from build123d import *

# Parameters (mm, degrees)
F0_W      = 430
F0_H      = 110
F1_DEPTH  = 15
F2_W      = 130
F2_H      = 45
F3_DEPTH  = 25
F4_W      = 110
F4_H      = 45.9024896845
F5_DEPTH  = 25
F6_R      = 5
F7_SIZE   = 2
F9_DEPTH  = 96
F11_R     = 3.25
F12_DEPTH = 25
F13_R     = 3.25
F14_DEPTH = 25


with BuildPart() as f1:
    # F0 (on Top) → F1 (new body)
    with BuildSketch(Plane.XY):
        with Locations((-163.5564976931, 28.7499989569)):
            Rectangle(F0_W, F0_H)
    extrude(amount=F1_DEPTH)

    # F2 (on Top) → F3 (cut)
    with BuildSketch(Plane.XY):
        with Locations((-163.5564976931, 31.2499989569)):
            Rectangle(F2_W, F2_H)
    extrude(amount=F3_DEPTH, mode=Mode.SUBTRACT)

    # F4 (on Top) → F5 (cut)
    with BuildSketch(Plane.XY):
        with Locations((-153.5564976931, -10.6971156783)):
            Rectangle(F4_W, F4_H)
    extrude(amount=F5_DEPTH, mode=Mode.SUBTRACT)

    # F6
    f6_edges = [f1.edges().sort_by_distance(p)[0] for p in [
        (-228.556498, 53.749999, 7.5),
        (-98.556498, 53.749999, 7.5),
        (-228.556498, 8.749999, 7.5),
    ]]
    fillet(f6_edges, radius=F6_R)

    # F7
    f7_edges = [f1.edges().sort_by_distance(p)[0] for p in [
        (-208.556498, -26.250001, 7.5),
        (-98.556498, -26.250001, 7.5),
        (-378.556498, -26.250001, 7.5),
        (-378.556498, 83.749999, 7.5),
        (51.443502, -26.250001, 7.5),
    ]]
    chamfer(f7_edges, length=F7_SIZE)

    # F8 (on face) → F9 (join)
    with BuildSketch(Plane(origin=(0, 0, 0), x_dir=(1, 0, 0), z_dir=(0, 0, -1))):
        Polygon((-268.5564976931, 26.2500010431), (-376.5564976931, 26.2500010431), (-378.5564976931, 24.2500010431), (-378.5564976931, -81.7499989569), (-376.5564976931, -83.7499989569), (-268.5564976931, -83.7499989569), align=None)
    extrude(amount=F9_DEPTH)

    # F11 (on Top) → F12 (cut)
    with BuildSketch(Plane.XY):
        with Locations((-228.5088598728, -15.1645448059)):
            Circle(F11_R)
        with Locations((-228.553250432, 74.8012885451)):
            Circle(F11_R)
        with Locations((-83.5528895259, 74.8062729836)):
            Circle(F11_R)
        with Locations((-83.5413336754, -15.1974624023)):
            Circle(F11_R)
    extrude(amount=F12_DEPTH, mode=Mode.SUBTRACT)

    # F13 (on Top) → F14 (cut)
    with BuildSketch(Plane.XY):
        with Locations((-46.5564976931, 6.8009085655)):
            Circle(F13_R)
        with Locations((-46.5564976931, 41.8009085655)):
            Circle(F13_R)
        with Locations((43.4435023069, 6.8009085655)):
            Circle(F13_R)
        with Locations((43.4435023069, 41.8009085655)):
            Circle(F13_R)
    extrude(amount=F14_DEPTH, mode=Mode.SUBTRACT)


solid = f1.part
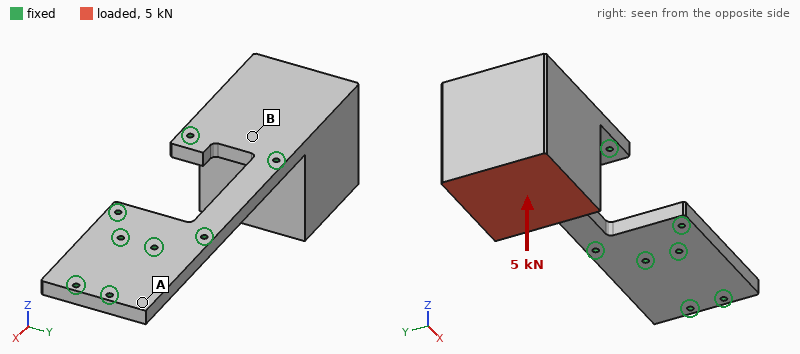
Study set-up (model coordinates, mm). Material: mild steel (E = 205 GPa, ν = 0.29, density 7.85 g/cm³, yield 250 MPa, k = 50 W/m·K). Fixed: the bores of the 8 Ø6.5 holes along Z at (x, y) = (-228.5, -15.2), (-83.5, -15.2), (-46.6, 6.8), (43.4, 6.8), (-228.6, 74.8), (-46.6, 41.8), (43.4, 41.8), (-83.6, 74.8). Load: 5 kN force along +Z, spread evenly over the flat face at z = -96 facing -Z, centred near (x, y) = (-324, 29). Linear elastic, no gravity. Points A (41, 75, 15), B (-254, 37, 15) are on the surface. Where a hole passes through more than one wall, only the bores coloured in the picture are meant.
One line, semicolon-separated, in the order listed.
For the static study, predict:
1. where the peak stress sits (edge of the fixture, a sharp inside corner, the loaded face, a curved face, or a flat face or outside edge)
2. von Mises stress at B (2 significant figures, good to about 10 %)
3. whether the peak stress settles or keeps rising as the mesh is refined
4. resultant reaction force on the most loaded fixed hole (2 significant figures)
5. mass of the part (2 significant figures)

edge of the fixture; 56 MPa; keeps rising; 2.8 kN; 14 kg
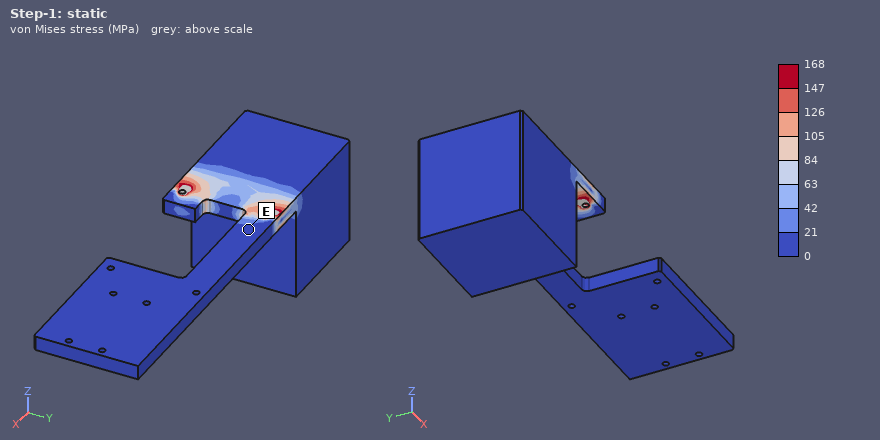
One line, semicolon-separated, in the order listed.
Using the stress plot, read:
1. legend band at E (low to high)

0 to 21 MPa
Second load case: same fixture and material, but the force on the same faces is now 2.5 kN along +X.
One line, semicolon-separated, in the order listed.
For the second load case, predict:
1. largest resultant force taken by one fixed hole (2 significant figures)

1.4 kN
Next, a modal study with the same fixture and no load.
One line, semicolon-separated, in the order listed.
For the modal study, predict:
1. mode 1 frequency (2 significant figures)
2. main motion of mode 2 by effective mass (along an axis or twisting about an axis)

160 Hz; along Y
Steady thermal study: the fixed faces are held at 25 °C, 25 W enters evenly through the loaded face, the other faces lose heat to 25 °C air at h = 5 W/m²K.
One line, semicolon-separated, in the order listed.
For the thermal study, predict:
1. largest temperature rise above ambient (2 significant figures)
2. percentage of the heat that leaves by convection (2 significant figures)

21 K; 24 %
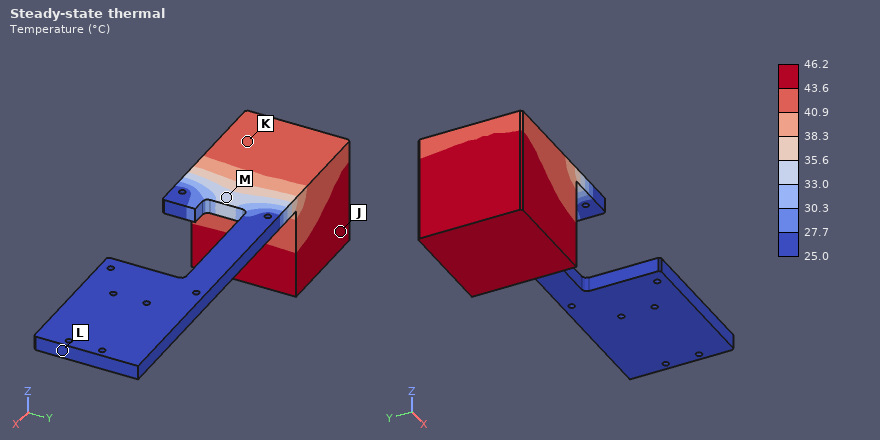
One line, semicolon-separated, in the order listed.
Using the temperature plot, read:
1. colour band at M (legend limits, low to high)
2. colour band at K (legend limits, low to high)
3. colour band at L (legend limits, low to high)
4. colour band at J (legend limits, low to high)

33.0 to 35.6 °C; 40.9 to 43.6 °C; 25.0 to 27.7 °C; 43.6 to 46.2 °C
